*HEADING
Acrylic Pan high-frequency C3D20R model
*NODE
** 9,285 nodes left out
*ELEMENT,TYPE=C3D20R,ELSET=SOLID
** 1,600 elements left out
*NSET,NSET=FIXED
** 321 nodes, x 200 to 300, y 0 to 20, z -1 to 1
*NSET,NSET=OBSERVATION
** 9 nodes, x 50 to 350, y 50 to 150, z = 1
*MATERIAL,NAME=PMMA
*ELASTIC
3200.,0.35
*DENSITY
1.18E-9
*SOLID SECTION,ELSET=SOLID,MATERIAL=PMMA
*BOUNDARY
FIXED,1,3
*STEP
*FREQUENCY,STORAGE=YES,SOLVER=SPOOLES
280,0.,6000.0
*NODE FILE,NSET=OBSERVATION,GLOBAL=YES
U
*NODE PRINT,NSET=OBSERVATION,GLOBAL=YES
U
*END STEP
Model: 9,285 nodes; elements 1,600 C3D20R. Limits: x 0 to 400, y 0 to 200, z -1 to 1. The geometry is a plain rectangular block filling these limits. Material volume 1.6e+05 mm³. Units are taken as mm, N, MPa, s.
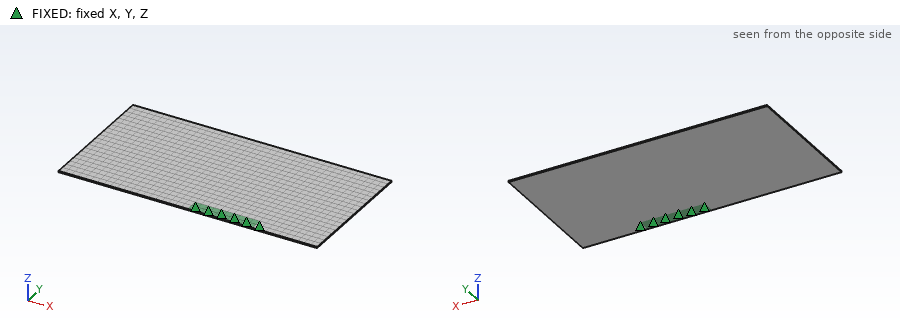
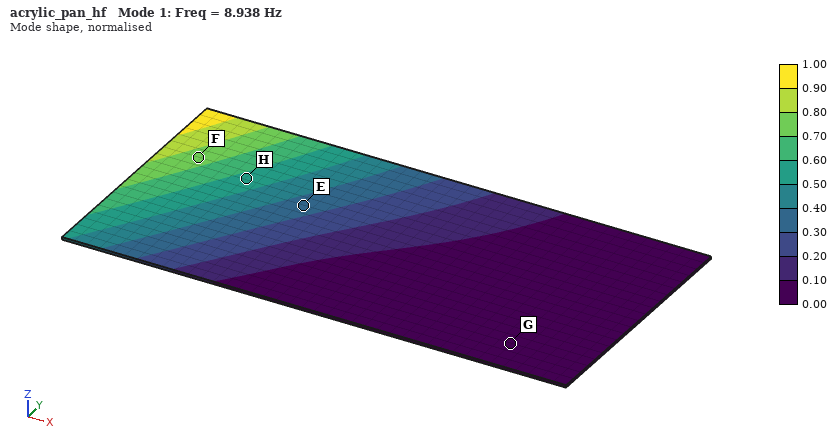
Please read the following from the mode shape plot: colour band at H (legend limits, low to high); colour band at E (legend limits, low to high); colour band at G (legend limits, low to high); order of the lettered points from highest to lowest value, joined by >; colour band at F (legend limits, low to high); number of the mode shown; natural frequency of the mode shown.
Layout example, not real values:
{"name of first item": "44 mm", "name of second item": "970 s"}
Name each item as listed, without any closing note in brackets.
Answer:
{"colour band at H": "0.50 to 0.60", "colour band at E": "0.30 to 0.40", "colour band at G": "0.00 to 0.10", "order of the lettered points from highest to lowest value, joined by >": "F > H > E > G", "colour band at F": "0.70 to 0.80", "number of the mode shown": "1", "natural frequency of the mode shown": "8.938 Hz"}
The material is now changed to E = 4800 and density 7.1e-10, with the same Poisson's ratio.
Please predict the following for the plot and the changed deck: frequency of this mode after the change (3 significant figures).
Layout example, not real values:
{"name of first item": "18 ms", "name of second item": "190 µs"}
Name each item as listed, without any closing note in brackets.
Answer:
{"frequency of this mode after the change": "14.1 Hz"}
